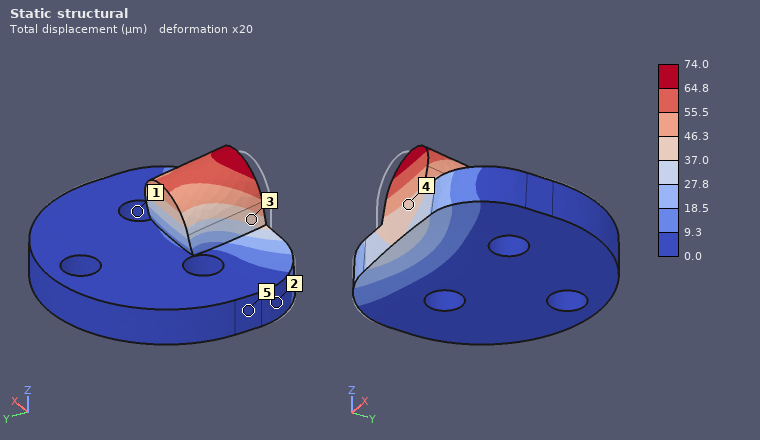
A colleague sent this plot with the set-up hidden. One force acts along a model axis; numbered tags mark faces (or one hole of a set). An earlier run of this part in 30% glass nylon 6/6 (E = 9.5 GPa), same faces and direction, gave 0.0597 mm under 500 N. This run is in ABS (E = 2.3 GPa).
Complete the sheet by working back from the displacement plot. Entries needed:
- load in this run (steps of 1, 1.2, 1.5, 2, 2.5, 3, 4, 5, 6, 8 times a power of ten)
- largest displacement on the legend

150 N
74.0 µm
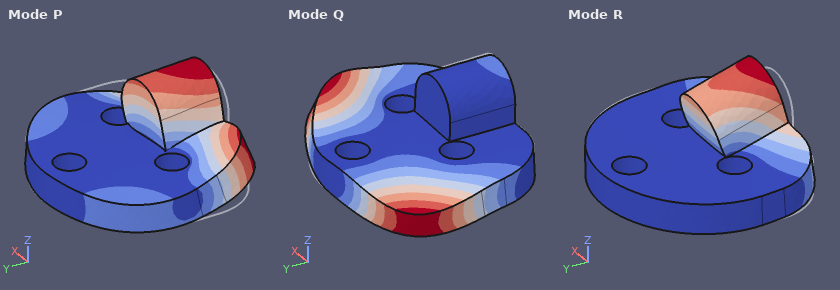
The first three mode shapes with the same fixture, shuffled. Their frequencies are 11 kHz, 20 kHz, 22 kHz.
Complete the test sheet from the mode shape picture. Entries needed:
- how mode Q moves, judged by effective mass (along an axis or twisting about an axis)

twisting about Y
